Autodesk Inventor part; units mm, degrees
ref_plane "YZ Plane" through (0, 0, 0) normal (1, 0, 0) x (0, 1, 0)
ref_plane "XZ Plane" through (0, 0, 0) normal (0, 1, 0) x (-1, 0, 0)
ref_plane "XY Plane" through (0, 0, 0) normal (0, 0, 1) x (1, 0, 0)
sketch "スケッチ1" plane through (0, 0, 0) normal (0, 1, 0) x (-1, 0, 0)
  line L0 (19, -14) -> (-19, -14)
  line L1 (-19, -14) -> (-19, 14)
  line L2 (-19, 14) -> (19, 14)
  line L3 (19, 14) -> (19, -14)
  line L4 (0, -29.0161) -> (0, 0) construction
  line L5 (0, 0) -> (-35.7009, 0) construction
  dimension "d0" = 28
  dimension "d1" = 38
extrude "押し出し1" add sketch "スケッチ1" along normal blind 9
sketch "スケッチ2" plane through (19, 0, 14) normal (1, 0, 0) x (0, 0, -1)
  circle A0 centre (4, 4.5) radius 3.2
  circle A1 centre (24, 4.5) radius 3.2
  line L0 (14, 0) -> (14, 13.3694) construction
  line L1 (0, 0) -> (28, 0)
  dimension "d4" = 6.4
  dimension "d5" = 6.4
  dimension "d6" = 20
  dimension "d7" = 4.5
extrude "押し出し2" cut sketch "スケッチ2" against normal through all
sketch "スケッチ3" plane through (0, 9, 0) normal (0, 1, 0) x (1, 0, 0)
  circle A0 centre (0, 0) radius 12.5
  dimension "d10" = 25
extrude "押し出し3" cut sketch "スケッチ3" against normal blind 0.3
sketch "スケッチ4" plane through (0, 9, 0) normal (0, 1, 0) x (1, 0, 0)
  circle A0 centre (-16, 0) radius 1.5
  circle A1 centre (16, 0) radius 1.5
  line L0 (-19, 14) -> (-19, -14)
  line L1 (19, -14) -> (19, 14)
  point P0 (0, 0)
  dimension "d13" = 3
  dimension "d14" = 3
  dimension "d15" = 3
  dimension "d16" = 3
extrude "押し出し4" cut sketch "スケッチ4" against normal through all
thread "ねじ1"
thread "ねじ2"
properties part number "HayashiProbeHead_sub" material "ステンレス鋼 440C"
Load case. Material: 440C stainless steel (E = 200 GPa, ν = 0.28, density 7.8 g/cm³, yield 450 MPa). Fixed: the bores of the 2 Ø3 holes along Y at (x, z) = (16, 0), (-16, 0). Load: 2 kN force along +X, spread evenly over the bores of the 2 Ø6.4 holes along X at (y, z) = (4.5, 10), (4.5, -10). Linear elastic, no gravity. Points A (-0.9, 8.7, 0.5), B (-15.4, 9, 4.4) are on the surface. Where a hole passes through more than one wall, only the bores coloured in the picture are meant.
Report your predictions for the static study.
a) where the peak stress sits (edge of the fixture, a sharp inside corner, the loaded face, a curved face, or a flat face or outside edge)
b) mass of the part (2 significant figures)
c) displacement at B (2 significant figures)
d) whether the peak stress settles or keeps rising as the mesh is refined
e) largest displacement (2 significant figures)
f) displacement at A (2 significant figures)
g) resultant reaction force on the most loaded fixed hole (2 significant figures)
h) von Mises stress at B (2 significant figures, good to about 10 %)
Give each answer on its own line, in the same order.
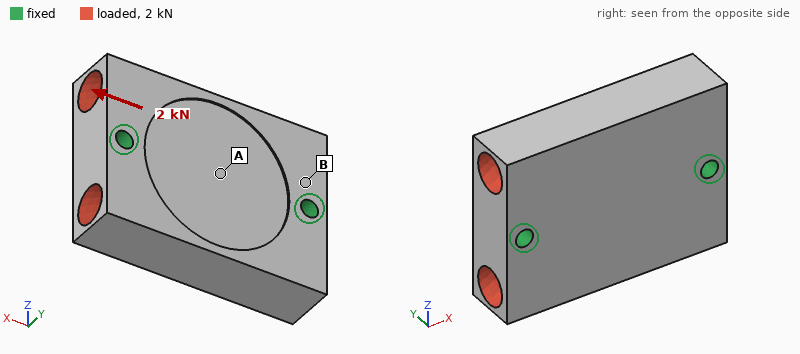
edge of the fixture
53 g
0.33 µm
keeps rising
1.2 µm
0.46 µm
1.0 kN
6.7 MPa
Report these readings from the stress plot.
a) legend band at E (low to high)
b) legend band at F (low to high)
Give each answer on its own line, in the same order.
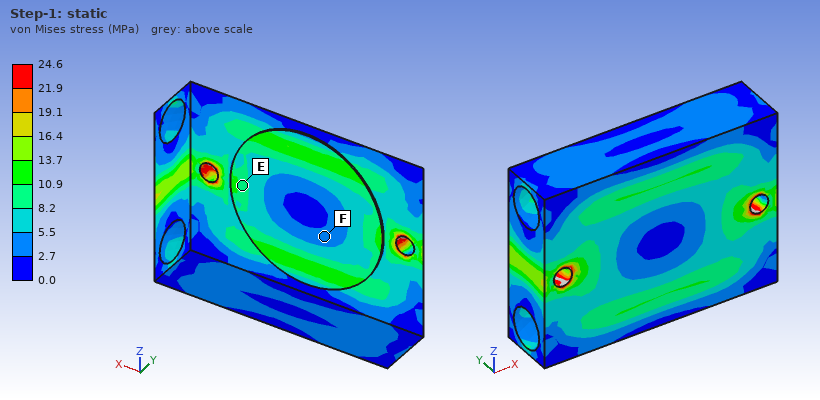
8.2 to 10.9 MPa
2.7 to 5.5 MPa
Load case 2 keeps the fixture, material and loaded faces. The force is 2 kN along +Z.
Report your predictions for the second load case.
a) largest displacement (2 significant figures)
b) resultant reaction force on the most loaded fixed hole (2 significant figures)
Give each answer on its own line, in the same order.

1.5 µm
1.0 kN
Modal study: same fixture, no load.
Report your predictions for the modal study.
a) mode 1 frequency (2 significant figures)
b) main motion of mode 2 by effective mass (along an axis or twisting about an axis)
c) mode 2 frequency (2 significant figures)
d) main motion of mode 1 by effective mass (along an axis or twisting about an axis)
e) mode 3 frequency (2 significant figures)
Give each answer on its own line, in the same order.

19 kHz
along Y
22 kHz
twisting about X
32 kHz
